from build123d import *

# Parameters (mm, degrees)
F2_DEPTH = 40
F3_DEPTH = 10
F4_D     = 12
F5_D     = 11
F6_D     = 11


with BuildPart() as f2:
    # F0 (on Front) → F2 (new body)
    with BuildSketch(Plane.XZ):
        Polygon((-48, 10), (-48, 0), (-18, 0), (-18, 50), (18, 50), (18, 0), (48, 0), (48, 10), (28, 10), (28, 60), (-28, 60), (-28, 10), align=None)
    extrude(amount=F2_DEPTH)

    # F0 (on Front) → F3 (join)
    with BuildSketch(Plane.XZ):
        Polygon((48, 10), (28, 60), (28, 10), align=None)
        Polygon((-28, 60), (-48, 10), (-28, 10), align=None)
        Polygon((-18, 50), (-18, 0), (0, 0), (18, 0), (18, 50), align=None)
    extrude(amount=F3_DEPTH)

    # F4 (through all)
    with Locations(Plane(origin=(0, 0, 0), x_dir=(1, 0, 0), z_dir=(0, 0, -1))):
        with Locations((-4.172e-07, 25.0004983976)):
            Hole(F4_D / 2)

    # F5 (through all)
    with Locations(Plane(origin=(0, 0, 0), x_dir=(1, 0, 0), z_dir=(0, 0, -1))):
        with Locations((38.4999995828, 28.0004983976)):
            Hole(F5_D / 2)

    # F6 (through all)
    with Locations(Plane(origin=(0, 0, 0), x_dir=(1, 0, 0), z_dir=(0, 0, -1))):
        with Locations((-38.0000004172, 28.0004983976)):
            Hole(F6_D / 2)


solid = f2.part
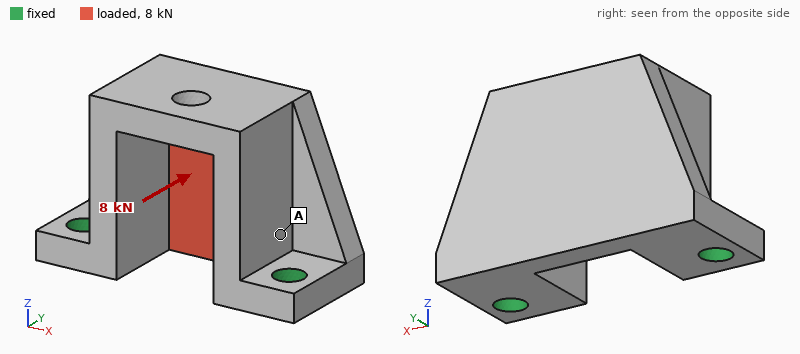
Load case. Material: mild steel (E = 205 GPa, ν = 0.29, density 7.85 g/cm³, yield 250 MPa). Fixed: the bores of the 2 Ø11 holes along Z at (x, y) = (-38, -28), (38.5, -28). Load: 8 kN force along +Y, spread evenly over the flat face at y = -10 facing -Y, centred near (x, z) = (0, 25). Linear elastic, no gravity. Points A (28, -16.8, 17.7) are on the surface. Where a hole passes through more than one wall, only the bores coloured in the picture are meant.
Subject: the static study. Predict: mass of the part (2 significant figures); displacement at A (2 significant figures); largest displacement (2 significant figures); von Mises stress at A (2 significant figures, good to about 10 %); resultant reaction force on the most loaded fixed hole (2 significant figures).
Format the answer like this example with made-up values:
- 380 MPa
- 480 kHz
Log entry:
- 810 g
- 16 µm
- 57 µm
- 19 MPa
- 4.5 kN
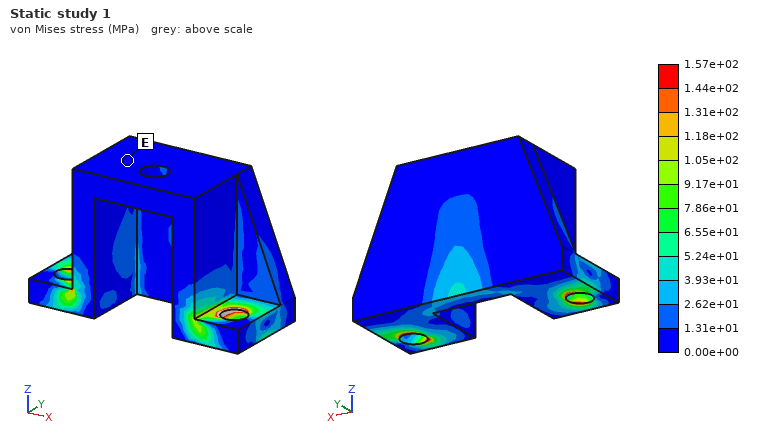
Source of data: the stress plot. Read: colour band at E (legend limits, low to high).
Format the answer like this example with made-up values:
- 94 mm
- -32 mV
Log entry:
- 0.00e+00 to 1.31e+01 MPa
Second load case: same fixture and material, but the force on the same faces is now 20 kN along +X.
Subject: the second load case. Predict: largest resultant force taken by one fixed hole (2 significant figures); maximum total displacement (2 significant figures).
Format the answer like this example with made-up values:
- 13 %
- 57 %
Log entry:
- 12 kN
- 44 µm
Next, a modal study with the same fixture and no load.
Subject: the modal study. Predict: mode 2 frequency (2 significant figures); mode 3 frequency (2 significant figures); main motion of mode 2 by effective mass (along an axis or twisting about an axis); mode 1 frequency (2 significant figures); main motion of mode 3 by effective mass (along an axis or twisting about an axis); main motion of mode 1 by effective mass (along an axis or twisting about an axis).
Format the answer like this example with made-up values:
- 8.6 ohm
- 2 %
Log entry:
- 3600 Hz
- 7400 Hz
- along X
- 2200 Hz
- along X
- along Y
